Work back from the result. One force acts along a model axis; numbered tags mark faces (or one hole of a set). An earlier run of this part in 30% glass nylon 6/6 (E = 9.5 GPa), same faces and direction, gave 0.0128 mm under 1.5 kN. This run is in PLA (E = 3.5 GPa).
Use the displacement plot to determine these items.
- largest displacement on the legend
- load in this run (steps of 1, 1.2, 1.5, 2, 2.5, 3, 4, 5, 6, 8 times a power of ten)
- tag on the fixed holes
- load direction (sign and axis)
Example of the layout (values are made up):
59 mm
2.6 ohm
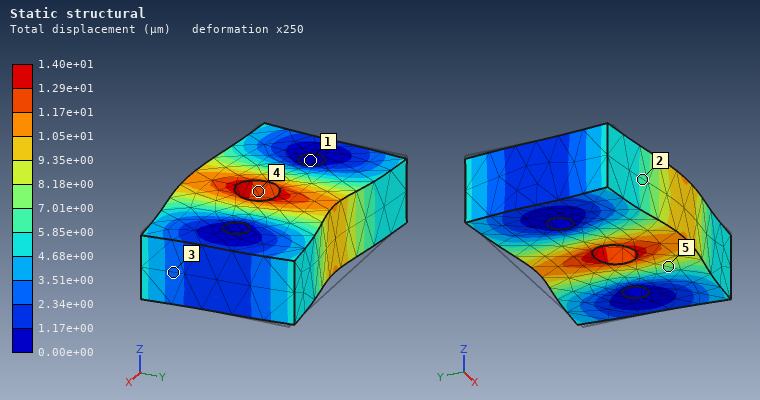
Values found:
1.40e+01 µm
600 N
1
-Y
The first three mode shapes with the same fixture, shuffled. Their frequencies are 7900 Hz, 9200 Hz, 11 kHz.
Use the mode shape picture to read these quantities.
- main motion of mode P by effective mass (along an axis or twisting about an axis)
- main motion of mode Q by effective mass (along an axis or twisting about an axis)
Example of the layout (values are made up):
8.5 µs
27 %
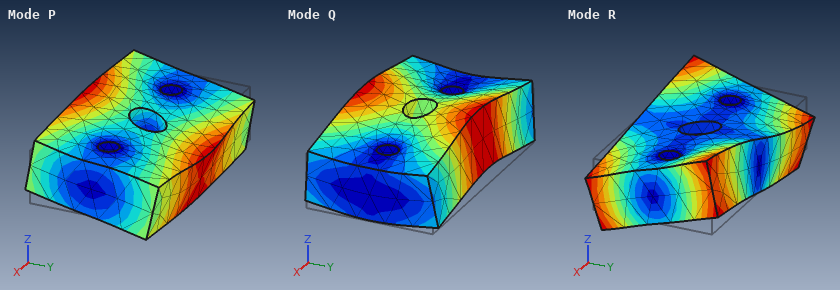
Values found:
twisting about X
along Z
